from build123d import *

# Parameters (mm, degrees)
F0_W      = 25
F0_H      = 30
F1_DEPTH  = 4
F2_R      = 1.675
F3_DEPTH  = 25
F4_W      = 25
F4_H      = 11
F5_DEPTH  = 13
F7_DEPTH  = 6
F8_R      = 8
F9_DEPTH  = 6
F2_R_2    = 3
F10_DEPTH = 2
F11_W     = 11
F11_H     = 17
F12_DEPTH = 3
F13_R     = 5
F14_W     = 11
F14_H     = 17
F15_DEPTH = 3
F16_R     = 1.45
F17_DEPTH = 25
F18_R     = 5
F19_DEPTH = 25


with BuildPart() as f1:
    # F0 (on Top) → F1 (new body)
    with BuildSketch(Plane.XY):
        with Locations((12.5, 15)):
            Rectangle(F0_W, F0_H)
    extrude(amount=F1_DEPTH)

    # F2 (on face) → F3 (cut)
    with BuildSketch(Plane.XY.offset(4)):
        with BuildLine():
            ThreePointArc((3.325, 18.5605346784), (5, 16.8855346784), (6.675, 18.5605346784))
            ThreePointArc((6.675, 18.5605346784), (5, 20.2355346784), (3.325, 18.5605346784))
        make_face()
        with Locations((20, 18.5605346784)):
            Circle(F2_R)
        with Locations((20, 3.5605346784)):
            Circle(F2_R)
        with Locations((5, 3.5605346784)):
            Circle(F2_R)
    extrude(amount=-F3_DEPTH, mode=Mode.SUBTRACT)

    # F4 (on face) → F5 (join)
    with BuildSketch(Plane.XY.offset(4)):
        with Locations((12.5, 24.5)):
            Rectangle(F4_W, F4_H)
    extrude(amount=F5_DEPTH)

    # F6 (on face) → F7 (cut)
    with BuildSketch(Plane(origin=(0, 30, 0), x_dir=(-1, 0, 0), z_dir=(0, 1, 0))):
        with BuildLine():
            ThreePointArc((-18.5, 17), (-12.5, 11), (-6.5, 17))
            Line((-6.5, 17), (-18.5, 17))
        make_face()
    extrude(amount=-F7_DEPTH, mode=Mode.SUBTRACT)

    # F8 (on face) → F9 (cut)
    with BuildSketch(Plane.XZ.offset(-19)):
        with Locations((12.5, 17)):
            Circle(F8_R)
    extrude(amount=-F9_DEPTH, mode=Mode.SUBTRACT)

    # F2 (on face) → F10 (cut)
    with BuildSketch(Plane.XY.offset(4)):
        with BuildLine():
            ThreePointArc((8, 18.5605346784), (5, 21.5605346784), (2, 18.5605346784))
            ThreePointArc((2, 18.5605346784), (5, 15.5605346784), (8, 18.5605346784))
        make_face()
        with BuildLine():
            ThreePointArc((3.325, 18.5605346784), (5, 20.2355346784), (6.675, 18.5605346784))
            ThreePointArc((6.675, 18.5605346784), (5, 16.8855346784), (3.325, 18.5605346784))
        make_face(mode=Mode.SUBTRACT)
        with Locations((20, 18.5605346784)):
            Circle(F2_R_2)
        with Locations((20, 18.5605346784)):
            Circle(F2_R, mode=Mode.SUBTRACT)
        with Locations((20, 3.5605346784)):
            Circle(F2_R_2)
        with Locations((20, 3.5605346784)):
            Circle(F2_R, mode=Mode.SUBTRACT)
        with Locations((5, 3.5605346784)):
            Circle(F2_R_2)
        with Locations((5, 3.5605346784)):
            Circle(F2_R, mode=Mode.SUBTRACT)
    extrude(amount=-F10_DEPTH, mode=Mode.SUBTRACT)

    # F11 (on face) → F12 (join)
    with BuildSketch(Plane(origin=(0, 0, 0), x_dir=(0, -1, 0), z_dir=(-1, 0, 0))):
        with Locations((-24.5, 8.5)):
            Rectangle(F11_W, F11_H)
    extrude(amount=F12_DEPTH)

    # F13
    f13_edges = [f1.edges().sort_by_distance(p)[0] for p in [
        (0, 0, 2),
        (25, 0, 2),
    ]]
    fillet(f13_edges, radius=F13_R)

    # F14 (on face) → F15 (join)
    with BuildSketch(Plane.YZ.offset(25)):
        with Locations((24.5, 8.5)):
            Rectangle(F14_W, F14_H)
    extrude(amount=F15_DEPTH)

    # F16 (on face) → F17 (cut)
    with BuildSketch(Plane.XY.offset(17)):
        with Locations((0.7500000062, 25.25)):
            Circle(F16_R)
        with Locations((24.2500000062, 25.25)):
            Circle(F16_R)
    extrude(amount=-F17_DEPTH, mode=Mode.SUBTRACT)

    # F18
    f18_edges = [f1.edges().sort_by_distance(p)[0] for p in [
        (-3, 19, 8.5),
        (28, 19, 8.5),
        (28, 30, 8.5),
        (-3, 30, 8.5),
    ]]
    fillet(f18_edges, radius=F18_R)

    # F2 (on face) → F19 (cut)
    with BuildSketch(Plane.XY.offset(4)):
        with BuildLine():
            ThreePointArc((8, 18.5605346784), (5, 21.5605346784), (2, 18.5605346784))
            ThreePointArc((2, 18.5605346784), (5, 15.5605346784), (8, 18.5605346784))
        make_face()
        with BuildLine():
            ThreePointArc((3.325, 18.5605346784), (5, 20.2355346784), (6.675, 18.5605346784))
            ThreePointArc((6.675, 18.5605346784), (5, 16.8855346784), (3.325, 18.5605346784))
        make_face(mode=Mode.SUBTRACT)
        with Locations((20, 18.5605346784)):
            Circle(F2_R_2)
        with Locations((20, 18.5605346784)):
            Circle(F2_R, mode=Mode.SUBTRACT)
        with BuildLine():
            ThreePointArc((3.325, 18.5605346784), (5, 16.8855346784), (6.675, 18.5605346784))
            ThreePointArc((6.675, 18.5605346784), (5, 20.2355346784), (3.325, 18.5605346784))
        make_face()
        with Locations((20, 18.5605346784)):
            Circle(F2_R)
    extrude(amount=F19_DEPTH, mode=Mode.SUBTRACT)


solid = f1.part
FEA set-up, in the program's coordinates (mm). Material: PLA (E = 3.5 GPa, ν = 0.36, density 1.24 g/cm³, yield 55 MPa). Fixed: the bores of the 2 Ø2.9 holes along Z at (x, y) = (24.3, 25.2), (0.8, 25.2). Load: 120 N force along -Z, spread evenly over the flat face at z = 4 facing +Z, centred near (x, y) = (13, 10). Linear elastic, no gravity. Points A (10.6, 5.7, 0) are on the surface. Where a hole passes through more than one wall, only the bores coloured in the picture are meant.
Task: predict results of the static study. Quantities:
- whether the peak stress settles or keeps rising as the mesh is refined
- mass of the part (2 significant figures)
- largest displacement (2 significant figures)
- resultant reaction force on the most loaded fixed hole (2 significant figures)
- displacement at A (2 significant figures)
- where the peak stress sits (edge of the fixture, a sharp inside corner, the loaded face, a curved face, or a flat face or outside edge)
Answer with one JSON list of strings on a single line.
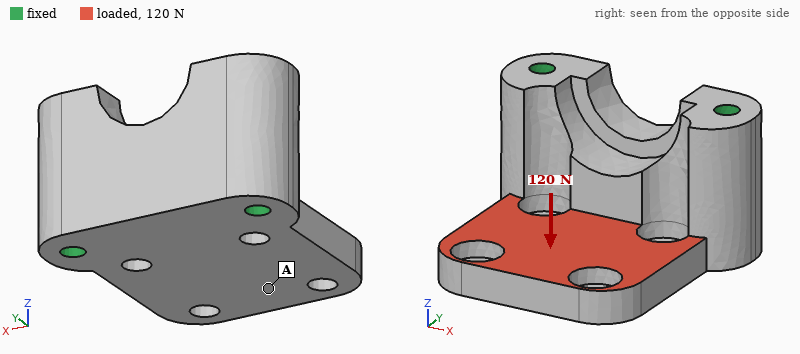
["keeps rising", "7.0 g", "0.46 mm", "60 N", "0.31 mm", "a sharp inside corner"]
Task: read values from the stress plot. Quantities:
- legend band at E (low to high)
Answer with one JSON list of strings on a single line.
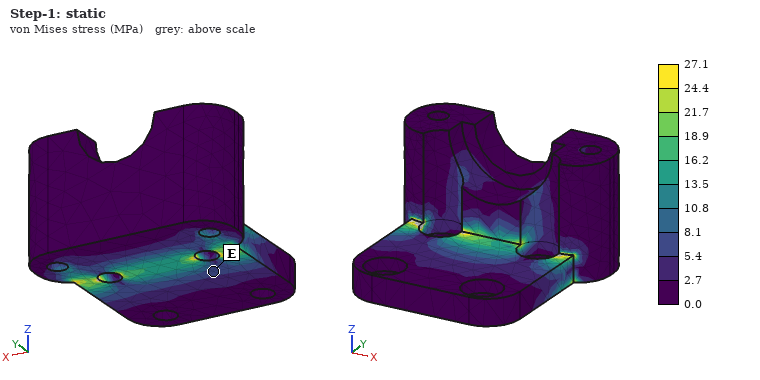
["5.4 to 8.1 MPa"]
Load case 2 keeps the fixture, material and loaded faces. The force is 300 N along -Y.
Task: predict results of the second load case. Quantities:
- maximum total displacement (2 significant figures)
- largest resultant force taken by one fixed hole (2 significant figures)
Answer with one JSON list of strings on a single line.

["0.27 mm", "150 N"]
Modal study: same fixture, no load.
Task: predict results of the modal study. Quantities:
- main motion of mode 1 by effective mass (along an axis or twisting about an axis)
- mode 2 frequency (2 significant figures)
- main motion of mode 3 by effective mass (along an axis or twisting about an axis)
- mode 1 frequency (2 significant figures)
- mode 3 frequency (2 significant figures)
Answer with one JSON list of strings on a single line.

["along Z", "4900 Hz", "along X", "2300 Hz", "7700 Hz"]
